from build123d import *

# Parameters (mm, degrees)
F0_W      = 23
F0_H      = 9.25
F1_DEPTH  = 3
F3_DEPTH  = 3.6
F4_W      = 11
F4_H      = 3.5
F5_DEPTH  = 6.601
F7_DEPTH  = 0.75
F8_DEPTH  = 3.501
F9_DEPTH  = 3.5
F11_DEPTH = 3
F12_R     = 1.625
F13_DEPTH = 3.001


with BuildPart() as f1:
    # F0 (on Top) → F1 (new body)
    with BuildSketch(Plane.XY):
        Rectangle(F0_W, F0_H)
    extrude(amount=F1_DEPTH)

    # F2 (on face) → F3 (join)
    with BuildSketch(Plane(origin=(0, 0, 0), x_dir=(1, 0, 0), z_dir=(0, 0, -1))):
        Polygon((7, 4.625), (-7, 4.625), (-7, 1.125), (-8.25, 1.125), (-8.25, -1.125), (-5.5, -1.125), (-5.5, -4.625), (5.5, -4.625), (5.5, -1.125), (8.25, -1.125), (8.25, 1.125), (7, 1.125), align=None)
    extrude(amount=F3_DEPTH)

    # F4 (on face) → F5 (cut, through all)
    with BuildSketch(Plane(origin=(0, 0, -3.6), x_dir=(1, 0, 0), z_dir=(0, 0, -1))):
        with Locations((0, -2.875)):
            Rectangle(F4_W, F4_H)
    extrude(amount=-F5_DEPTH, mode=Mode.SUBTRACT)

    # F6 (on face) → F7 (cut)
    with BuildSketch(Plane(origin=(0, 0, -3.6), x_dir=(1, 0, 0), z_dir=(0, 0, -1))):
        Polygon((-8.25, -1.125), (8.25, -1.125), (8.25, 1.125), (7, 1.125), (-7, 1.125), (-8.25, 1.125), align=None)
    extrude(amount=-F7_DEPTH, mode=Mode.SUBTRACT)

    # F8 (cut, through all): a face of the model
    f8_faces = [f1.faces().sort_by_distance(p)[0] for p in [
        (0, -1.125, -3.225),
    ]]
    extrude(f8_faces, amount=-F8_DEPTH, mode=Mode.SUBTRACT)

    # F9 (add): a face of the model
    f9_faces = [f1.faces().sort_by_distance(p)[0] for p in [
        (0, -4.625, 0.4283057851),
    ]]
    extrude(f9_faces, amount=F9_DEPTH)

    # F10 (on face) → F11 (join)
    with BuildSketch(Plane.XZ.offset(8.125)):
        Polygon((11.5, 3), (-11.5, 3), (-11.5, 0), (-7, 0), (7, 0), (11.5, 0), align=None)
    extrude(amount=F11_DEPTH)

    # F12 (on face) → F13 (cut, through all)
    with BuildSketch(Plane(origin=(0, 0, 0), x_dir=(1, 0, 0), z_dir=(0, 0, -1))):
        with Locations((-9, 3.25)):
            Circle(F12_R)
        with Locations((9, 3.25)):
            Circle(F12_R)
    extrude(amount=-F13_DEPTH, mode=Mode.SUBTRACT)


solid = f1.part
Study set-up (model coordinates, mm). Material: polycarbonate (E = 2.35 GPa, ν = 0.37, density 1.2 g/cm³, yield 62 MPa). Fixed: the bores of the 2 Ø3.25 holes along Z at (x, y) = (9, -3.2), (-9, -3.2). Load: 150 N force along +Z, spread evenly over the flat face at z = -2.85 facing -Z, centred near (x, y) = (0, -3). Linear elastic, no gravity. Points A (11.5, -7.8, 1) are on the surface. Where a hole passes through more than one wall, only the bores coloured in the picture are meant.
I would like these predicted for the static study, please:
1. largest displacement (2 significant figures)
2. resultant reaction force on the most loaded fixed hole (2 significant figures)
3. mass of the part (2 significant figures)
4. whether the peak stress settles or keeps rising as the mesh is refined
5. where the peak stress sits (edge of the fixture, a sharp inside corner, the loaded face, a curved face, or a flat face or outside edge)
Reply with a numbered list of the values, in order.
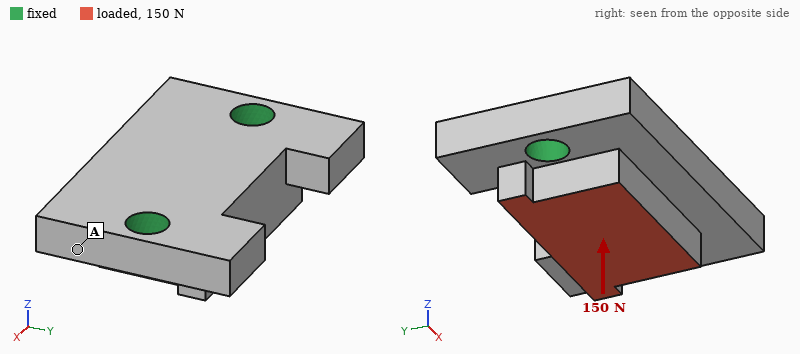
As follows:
1. 28 µm
2. 83 N
3. 1.6 g
4. keeps rising
5. edge of the fixture
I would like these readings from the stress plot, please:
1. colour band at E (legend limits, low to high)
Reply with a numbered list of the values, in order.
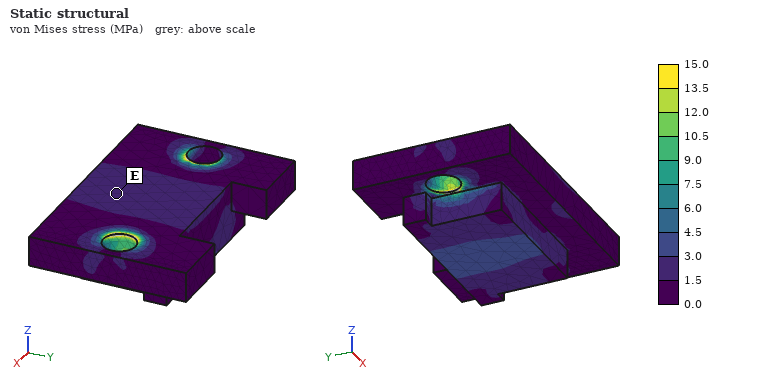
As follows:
1. 1.5 to 3.0 MPa
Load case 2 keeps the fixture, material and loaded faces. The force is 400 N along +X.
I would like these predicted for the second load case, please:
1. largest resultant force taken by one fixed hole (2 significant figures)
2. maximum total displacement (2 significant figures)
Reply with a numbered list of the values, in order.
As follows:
1. 230 N
2. 39 µm
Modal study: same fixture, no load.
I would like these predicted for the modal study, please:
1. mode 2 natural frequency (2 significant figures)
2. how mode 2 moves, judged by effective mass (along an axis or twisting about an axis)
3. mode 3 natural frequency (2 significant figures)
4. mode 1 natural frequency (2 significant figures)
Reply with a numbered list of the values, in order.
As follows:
1. 13 kHz
2. along Z
3. 16 kHz
4. 8700 Hz
